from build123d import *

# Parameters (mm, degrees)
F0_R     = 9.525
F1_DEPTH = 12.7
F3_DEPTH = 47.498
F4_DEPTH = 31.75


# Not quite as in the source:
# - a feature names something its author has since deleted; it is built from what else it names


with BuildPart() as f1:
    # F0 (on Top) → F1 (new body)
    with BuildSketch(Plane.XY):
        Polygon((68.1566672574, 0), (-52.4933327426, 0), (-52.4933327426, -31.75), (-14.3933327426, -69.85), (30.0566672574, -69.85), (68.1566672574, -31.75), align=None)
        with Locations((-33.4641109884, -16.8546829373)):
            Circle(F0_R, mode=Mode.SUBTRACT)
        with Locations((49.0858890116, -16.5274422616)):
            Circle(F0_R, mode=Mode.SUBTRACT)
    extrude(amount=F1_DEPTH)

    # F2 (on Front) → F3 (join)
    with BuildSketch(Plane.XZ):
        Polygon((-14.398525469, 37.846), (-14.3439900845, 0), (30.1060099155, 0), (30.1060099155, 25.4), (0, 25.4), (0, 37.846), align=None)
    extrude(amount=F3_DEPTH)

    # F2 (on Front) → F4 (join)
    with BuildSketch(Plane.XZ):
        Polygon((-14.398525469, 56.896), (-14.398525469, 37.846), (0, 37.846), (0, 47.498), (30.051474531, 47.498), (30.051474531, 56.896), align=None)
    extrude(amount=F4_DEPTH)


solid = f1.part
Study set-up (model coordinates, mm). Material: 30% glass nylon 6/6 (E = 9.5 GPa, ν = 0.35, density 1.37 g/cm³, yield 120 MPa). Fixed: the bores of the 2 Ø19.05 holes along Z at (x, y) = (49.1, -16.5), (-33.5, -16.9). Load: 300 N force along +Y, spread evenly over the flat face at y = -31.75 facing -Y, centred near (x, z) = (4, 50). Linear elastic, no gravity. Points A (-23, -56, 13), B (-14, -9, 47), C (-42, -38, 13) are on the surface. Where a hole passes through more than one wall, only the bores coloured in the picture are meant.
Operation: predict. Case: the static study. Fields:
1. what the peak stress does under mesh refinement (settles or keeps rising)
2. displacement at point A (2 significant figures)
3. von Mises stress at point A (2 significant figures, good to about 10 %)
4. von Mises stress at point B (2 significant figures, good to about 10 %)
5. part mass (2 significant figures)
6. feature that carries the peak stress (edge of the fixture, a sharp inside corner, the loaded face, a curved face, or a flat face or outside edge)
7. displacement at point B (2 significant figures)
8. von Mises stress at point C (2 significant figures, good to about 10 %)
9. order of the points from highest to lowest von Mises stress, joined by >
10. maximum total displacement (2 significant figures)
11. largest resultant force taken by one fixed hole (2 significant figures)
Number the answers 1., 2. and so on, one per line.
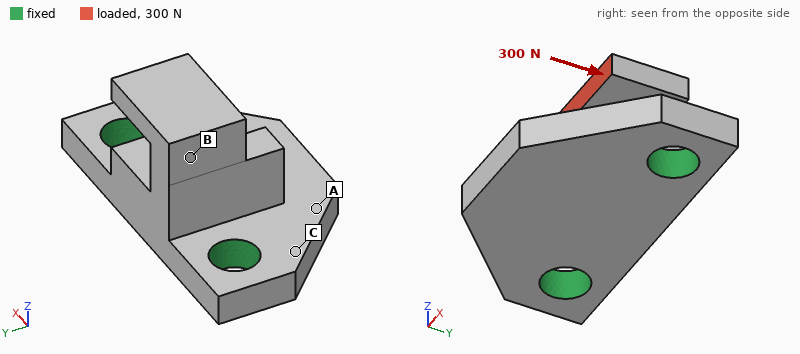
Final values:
1. keeps rising
2. 26 µm
3. 0.55 MPa
4. 1.2 MPa
5. 180 g
6. edge of the fixture
7. 40 µm
8. 1.8 MPa
9. C > B > A
10. 97 µm
11. 170 N
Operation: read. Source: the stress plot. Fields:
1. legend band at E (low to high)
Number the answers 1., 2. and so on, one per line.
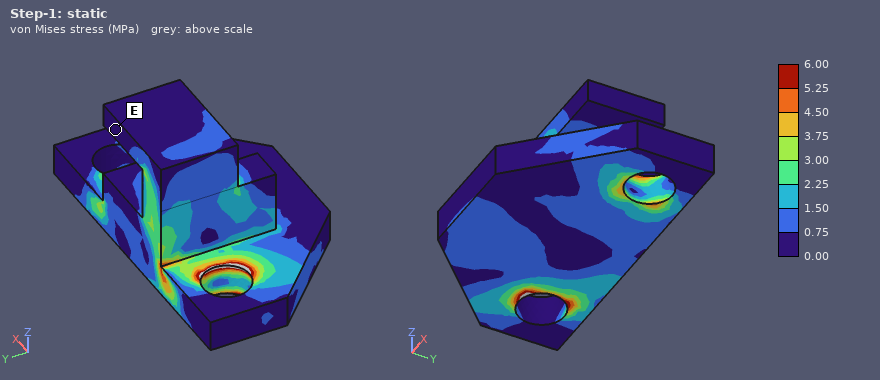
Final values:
1. 0.00 to 0.75 MPa
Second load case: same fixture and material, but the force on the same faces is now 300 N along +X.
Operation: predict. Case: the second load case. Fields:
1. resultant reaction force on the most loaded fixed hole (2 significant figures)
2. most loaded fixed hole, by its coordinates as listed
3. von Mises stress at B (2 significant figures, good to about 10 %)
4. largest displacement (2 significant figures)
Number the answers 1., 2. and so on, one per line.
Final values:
1. 310 N
2. (49.1, -16.5)
3. 2.3 MPa
4. 0.11 mm
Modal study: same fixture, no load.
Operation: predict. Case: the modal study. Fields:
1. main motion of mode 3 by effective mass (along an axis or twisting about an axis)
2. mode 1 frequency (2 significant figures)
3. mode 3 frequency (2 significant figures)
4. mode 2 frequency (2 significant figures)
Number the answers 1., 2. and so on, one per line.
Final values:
1. along Z
2. 1700 Hz
3. 3000 Hz
4. 1900 Hz
